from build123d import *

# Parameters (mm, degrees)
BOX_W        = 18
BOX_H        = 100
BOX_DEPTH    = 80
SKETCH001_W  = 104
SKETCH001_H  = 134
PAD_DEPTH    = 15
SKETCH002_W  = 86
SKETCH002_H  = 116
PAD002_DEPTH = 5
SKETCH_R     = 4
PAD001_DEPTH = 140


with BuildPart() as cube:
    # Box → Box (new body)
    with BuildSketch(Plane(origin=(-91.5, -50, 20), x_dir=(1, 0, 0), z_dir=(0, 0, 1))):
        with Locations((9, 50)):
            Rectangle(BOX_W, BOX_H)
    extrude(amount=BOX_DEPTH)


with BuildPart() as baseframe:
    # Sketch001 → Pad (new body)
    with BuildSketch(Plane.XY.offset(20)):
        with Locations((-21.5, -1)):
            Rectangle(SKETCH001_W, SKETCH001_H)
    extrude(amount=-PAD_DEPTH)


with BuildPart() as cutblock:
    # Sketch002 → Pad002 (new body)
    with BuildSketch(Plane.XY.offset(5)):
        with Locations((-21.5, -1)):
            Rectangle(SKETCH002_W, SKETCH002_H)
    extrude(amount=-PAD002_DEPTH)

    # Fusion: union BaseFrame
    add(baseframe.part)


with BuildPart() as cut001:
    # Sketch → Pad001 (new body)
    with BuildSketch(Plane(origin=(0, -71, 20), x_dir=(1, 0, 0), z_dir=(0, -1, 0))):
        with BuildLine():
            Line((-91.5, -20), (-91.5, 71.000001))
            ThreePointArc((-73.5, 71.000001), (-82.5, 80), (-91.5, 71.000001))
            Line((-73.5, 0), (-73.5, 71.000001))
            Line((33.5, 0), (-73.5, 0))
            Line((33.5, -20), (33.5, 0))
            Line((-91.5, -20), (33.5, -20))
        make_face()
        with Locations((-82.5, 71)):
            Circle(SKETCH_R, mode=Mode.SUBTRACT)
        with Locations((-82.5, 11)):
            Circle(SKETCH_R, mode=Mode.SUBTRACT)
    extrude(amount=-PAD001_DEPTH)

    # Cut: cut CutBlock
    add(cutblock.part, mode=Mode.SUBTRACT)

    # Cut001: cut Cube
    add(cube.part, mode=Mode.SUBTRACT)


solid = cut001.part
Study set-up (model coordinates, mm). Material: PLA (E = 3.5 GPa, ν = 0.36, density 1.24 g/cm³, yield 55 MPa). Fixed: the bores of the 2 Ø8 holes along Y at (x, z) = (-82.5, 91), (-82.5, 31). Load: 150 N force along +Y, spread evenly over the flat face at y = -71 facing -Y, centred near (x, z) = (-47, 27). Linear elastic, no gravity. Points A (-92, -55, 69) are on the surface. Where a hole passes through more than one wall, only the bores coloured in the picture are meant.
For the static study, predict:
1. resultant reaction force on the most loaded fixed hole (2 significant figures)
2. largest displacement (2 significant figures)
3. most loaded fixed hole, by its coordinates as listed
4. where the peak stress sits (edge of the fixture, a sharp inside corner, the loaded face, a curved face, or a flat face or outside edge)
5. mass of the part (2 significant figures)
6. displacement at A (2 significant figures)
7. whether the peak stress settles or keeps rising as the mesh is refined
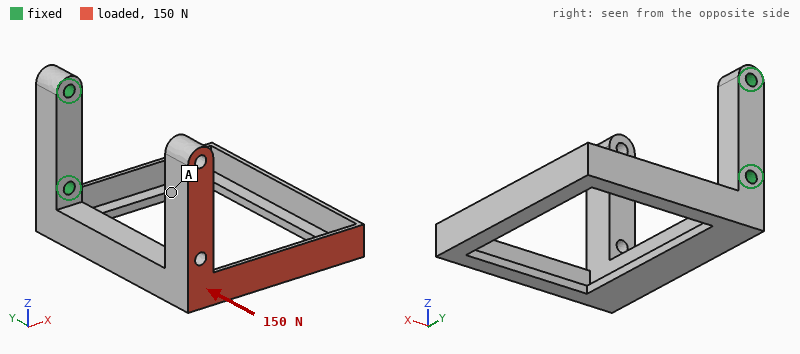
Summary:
150 N
2.3 mm
(-82.5, 31)
edge of the fixture
180 g
0.98 mm
keeps rising
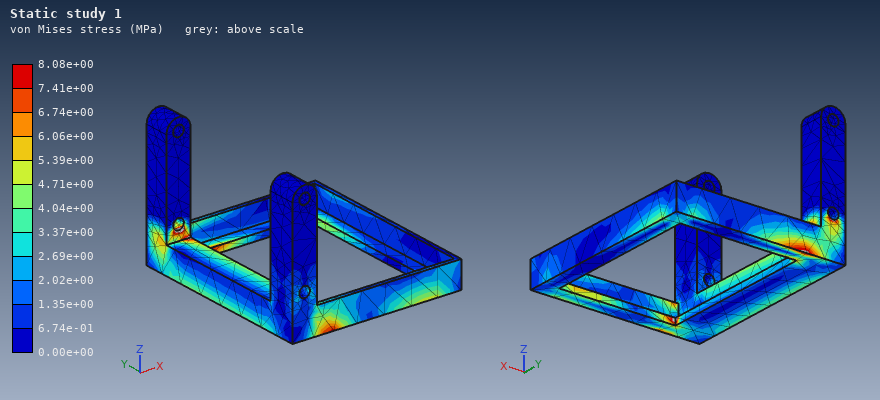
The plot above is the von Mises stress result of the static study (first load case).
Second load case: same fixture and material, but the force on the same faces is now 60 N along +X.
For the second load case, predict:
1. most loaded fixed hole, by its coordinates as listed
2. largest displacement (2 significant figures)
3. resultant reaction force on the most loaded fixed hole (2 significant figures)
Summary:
(-82.5, 31)
1.9 mm
61 N
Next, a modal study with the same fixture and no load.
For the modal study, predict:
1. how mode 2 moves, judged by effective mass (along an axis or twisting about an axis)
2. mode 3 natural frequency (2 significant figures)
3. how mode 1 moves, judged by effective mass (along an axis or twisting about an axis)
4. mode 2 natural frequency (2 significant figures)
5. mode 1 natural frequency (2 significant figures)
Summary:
along Z
170 Hz
along X
110 Hz
110 Hz
